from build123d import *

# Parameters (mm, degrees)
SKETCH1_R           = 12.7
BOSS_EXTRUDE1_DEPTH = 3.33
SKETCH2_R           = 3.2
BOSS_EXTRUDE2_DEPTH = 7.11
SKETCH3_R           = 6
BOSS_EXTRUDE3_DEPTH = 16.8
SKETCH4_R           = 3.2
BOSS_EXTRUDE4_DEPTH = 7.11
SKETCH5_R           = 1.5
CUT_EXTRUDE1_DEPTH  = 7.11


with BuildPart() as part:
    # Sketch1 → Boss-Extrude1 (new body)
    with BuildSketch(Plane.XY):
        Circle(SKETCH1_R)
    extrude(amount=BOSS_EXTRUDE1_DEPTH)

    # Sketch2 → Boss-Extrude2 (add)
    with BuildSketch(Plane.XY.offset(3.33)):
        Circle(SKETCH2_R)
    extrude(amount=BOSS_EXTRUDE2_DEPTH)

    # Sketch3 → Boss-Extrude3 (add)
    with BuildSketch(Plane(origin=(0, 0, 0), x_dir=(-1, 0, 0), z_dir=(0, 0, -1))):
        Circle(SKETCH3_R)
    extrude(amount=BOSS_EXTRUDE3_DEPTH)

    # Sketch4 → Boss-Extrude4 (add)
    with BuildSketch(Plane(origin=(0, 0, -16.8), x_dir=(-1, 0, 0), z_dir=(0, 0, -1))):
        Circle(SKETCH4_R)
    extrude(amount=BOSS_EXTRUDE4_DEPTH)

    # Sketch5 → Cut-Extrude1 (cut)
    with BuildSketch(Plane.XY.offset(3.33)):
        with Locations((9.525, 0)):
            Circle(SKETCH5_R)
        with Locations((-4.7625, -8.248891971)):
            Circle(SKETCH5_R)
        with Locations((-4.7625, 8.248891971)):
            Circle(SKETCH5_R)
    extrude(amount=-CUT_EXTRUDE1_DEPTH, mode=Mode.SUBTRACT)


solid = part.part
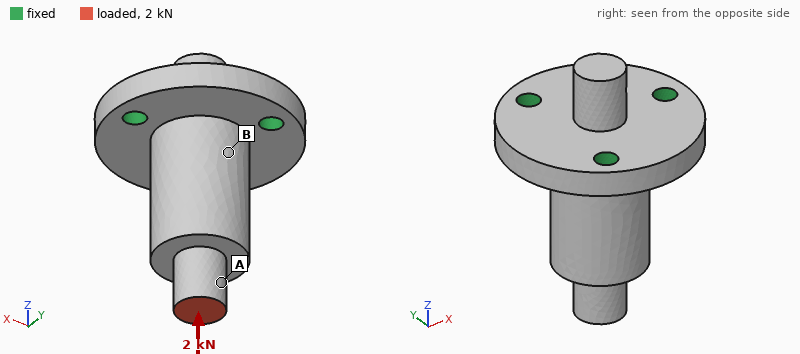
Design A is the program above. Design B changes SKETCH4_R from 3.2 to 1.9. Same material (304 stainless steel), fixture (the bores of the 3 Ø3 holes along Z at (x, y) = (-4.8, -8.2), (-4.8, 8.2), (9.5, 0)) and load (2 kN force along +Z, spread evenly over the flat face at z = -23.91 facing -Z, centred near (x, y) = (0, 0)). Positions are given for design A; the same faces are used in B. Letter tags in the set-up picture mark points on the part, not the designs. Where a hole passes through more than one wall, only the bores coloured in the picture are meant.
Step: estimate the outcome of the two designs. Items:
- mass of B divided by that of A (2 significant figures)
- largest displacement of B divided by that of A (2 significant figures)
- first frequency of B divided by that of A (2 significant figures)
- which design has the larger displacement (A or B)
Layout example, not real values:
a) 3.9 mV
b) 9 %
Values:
a) 0.96
b) 1.8
c) 1.1
d) B
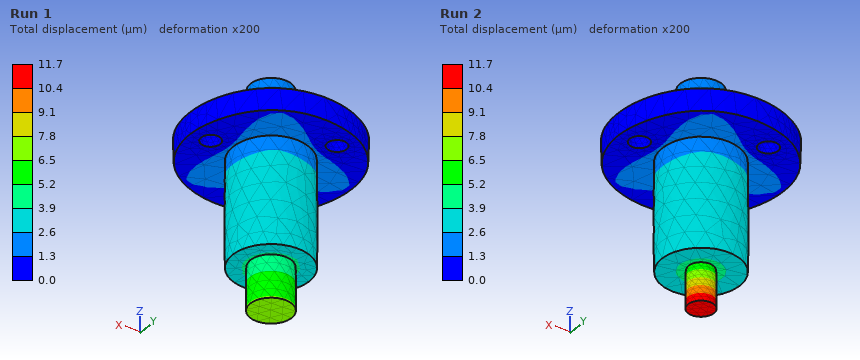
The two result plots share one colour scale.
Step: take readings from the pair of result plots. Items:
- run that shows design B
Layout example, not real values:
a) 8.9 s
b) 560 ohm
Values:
a) Run 2
